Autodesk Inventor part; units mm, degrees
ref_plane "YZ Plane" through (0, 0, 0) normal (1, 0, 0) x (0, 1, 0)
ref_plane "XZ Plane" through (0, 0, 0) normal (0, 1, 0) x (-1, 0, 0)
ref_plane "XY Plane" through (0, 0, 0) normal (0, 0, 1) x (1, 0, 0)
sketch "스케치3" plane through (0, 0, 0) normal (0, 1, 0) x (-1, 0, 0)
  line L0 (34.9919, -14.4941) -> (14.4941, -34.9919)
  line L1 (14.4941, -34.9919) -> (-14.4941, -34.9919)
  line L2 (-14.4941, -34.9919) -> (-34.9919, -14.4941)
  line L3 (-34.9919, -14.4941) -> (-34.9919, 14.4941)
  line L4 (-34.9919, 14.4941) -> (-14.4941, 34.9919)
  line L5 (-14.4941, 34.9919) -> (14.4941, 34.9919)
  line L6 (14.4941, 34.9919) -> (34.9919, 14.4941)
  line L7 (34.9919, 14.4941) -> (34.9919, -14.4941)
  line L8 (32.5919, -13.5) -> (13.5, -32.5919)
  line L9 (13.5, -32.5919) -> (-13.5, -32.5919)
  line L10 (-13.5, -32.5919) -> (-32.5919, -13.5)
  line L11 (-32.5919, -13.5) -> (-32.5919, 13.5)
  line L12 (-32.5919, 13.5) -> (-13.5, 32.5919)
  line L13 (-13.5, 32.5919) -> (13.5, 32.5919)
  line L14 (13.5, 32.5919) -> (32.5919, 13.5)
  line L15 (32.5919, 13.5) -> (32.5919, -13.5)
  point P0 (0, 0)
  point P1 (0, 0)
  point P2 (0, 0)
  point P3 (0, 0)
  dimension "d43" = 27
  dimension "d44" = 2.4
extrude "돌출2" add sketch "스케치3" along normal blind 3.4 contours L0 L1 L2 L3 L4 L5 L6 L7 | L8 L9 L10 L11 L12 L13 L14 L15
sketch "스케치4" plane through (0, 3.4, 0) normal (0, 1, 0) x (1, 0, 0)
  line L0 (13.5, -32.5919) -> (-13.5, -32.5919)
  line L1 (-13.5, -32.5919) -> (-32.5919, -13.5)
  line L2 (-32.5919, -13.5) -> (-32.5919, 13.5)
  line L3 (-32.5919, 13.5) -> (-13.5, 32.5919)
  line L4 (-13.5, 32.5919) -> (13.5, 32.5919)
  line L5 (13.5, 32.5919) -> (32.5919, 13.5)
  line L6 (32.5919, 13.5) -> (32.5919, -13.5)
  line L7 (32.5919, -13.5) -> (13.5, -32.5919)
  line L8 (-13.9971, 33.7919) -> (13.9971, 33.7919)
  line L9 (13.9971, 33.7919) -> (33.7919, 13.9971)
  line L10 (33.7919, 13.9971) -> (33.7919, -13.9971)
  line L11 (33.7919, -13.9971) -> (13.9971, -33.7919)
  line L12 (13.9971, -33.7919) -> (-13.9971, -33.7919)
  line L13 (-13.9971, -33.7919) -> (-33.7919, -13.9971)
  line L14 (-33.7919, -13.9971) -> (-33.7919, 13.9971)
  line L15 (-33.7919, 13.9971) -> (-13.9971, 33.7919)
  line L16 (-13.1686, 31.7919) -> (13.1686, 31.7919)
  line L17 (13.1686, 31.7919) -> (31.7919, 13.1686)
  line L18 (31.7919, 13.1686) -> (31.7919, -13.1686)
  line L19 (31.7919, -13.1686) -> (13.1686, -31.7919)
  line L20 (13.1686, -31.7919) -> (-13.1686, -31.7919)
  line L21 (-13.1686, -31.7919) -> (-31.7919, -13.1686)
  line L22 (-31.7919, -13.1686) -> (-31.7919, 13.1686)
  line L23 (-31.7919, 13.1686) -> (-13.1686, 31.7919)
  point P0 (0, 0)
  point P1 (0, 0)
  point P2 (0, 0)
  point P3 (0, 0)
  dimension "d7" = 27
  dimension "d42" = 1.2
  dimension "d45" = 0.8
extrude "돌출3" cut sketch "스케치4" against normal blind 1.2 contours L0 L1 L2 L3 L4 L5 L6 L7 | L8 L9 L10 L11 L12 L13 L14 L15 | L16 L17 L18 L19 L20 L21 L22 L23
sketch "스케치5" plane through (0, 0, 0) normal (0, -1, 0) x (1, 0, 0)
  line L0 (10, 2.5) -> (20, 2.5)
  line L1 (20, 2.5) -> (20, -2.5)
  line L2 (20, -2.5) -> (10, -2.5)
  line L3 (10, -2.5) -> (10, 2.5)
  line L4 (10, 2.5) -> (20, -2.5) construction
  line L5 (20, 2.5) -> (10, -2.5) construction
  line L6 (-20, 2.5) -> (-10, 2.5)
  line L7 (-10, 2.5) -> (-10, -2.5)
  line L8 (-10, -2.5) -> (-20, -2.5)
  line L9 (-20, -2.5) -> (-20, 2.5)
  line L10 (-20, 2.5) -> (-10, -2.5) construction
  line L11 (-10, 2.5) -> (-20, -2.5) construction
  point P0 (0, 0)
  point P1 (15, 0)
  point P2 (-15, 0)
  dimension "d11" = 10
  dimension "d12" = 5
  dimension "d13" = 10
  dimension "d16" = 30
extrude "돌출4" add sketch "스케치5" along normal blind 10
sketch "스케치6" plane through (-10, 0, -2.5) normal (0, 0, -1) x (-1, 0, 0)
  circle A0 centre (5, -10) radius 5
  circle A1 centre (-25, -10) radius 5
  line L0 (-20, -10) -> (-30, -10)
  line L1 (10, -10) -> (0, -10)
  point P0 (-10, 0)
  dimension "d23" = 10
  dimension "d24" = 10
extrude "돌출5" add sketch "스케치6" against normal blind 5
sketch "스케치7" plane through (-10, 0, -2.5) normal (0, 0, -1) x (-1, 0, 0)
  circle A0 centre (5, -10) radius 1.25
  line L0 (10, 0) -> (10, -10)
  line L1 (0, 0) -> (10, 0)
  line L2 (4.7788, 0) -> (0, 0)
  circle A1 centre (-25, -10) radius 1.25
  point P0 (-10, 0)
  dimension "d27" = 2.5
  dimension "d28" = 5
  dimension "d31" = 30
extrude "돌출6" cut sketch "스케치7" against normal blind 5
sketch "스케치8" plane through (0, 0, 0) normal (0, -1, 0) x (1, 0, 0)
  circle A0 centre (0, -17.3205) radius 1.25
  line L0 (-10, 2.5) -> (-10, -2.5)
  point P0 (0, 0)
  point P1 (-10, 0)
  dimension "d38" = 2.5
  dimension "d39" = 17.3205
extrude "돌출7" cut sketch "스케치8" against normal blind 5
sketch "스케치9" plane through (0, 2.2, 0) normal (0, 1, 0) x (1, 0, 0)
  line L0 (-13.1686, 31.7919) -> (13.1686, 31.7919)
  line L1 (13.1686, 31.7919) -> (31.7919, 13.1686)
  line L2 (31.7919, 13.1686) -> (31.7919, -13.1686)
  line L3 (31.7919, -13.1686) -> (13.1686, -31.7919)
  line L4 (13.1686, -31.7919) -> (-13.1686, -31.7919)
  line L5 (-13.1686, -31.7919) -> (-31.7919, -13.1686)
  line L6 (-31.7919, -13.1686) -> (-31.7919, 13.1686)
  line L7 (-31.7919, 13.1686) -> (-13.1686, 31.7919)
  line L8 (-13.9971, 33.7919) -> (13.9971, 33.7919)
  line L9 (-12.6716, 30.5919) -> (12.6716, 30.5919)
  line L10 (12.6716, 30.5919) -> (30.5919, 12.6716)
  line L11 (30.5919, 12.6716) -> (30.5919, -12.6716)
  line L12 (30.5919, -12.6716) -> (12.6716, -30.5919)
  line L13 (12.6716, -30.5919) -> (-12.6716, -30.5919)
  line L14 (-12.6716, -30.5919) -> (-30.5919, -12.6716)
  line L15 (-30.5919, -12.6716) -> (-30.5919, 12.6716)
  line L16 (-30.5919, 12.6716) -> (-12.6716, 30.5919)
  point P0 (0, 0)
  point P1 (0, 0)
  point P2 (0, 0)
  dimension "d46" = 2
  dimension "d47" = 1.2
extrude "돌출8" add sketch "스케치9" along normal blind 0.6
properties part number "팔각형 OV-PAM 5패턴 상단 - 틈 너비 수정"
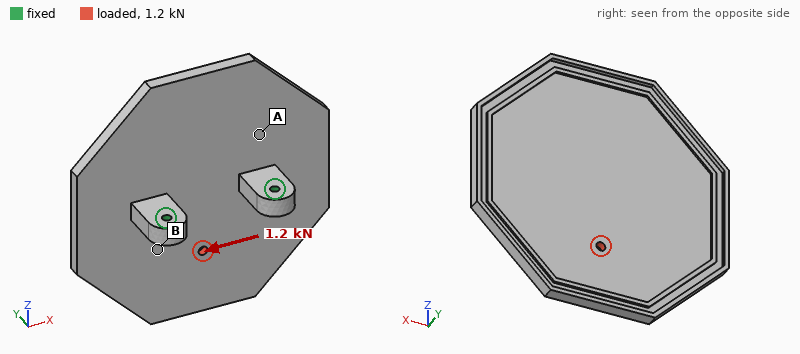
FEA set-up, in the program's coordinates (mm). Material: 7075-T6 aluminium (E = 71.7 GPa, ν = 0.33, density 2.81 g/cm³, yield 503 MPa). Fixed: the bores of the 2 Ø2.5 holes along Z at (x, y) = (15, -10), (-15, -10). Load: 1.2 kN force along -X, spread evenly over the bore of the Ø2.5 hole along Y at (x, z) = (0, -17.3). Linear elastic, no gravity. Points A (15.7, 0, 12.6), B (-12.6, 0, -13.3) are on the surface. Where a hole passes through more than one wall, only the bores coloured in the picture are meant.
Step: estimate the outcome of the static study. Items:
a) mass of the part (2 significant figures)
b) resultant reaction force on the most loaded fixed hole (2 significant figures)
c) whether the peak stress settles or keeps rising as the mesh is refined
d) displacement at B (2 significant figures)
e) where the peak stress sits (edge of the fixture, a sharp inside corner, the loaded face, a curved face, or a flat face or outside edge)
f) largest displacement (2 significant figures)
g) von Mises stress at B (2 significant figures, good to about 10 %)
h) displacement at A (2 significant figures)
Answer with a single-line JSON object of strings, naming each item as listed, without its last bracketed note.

{"mass of the part": "30 g", "resultant reaction force on the most loaded fixed hole": "840 N", "whether the peak stress settles or keeps rising as the mesh is refined": "keeps rising", "displacement at B": "0.072 mm", "where the peak stress sits": "edge of the fixture", "largest displacement": "0.12 mm", "von Mises stress at B": "37 MPa", "displacement at A": "0.046 mm"}
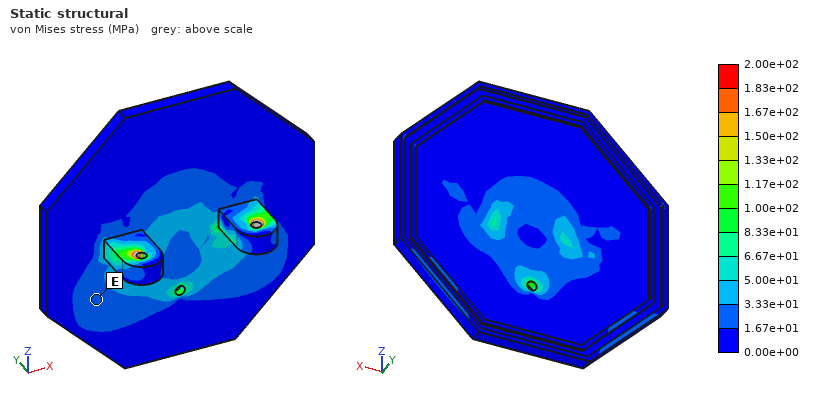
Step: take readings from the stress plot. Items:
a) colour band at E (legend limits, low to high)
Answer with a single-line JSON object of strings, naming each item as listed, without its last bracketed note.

{"colour band at E": "1.67e+01 to 3.33e+01 MPa"}
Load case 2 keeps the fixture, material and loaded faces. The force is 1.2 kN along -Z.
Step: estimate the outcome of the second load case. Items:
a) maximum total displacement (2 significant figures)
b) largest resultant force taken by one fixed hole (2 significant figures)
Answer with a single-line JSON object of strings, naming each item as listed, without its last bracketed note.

{"maximum total displacement": "0.20 mm", "largest resultant force taken by one fixed hole": "600 N"}
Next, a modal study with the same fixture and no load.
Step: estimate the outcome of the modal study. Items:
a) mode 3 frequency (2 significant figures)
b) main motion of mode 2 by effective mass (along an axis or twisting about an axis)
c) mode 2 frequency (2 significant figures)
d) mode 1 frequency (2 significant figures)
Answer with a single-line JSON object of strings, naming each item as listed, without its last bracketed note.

{"mode 3 frequency": "2600 Hz", "main motion of mode 2 by effective mass": "along Y", "mode 2 frequency": "1900 Hz", "mode 1 frequency": "1300 Hz"}
